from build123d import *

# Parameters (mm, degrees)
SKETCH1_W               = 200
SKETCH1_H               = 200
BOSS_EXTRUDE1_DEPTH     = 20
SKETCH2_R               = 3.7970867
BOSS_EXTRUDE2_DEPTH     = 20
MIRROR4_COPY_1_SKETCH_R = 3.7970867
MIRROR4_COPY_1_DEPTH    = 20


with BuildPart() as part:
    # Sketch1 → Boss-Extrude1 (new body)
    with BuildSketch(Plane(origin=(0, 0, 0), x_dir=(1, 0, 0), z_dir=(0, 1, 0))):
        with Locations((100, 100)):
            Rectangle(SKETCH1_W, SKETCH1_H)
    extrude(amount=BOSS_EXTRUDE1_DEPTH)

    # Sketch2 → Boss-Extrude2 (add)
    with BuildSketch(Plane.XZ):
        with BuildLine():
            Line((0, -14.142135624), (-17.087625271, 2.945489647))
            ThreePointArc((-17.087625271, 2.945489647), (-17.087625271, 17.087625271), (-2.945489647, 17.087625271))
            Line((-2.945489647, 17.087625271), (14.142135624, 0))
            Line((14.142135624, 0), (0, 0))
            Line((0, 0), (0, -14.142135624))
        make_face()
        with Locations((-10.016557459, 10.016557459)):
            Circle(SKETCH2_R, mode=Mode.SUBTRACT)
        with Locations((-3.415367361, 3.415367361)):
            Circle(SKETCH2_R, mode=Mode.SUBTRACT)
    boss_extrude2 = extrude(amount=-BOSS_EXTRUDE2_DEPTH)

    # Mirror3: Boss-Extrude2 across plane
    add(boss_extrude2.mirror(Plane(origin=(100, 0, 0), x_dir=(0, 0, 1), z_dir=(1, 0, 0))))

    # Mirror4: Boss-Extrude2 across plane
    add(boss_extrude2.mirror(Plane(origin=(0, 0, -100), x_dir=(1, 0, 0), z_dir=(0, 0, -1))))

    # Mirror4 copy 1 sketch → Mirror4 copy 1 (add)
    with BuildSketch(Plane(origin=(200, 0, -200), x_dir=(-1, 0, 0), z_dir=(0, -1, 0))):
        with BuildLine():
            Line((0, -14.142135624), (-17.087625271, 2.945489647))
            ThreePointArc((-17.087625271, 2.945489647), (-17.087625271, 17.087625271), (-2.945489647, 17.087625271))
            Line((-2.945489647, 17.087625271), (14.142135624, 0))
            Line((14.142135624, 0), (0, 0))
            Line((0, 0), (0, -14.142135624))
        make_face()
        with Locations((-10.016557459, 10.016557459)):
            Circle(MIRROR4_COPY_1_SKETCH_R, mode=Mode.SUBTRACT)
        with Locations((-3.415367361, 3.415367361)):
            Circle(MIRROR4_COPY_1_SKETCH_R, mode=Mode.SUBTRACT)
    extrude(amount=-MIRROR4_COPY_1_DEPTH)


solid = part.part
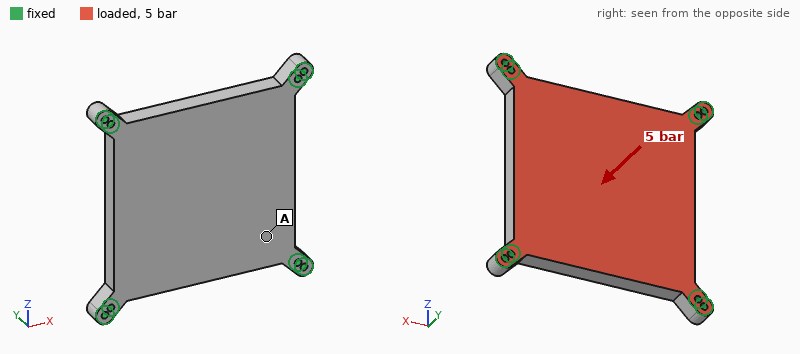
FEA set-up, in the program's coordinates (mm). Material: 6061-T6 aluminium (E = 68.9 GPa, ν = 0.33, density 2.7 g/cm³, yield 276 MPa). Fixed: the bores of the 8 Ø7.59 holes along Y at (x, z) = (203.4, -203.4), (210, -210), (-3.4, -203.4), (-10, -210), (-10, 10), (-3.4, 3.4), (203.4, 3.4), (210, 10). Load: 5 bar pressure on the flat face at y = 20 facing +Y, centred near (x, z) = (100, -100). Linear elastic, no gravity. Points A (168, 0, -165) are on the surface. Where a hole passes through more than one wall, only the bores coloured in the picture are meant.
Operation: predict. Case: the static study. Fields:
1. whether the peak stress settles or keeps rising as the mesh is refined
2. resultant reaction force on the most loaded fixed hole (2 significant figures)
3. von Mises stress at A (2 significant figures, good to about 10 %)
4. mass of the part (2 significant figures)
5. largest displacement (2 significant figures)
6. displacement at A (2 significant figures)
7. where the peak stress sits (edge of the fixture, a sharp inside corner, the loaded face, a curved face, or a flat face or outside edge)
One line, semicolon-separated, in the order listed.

keeps rising; 6.0 kN; 13 MPa; 2.3 kg; 0.21 mm; 0.11 mm; edge of the fixture
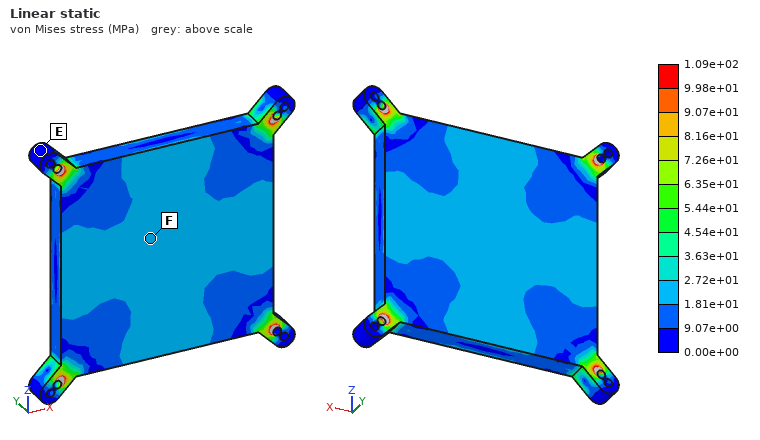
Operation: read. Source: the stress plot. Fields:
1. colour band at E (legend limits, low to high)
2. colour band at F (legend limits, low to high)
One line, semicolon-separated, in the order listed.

0.00e+00 to 9.07e+00 MPa; 1.81e+01 to 2.72e+01 MPa
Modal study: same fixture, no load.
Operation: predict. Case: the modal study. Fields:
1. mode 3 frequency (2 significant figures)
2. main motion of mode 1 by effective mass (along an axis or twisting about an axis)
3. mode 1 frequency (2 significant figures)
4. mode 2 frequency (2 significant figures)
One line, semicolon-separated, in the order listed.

2200 Hz; along Y; 1200 Hz; 2200 Hz
